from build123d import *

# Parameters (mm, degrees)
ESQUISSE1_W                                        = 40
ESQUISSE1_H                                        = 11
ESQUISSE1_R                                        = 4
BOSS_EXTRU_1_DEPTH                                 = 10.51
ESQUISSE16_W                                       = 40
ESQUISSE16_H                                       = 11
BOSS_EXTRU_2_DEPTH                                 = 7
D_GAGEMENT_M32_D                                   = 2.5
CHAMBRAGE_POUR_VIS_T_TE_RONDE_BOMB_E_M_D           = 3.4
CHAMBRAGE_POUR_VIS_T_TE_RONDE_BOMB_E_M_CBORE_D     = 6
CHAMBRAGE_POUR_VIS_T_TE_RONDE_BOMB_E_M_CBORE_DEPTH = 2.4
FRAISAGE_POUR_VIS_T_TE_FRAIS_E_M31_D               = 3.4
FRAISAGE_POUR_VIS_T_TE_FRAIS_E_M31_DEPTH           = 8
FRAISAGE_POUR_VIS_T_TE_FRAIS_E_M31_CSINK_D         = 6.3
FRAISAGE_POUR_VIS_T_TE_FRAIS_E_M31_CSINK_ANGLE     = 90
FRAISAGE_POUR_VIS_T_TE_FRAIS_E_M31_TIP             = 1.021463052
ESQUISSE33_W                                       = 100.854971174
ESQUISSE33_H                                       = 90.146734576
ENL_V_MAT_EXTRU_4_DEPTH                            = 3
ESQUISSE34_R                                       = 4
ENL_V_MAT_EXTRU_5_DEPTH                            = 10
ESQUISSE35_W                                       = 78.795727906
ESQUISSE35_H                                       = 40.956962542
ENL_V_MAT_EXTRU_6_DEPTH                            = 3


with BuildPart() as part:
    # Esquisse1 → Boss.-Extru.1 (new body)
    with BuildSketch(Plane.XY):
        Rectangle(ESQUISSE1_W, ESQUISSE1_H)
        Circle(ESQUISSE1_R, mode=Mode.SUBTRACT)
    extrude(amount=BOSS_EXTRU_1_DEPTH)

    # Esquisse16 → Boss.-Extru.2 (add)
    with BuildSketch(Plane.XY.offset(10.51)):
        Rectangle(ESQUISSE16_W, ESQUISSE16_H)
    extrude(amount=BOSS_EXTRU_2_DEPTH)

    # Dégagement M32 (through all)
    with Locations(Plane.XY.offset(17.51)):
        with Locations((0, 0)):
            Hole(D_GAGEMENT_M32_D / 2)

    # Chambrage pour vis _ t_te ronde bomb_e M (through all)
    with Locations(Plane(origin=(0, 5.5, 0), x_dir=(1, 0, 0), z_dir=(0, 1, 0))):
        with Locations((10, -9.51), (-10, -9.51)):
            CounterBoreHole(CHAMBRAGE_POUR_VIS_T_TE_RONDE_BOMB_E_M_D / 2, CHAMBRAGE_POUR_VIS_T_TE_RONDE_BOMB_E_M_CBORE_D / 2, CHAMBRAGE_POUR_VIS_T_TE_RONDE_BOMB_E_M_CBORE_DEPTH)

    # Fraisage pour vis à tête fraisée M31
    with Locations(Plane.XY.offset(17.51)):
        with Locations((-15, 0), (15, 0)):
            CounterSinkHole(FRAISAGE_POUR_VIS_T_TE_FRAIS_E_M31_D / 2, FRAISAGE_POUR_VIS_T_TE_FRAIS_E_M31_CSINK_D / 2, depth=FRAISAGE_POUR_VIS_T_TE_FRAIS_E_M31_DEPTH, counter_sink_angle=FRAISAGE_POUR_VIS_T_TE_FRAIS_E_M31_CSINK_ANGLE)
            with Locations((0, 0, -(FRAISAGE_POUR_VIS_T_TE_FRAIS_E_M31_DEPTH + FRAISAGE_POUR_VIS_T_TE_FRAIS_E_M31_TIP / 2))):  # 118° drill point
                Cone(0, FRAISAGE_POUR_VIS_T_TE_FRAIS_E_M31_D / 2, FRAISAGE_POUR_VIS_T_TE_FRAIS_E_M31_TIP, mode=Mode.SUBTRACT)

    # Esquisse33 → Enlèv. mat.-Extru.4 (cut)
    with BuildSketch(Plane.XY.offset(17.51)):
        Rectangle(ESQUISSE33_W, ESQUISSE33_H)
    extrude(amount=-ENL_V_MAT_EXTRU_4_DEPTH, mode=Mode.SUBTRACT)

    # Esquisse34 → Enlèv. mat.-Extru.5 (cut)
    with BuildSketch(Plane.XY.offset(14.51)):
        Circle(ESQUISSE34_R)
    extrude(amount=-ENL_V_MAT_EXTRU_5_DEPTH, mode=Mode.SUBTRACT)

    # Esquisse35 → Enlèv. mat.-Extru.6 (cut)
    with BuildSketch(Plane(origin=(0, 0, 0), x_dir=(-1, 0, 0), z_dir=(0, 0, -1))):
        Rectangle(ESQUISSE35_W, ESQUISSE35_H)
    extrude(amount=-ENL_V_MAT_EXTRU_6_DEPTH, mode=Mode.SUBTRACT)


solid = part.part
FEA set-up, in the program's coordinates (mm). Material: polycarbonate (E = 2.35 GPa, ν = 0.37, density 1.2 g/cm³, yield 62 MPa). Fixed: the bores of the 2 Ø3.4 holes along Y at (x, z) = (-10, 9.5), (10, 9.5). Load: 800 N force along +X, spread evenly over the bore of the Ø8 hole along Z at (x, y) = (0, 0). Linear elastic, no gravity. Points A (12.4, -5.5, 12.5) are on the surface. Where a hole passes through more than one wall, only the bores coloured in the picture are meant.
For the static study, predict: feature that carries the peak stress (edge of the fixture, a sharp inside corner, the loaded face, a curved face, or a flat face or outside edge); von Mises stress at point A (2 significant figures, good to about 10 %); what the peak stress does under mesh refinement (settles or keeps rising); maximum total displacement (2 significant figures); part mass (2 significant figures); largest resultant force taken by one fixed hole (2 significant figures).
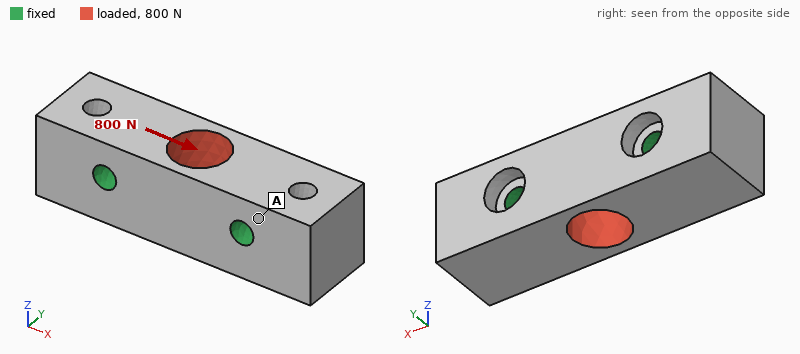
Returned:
edge of the fixture
1.5 MPa
keeps rising
24 µm
4.9 g
400 N
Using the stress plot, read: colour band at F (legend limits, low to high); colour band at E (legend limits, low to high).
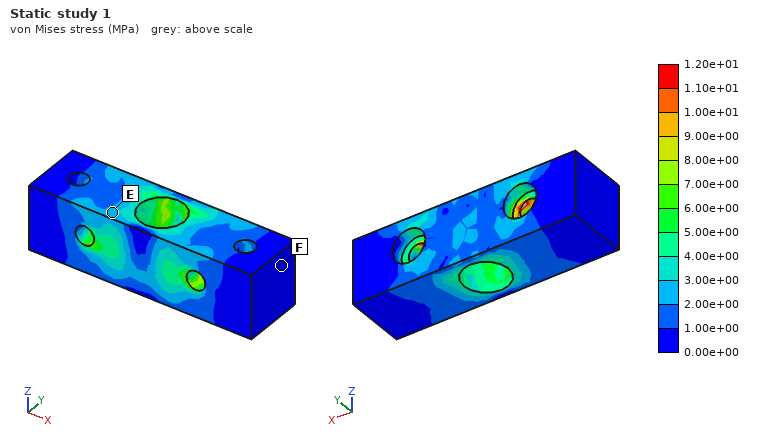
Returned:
0.00e+00 to 1.00e+00 MPa
2.00e+00 to 3.00e+00 MPa
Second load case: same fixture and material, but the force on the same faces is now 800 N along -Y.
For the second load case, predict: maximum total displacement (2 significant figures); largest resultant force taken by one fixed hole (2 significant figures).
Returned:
76 µm
400 N
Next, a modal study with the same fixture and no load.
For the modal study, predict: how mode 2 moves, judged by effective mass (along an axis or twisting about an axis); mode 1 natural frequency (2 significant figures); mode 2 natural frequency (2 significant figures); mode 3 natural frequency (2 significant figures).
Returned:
twisting about Y
9800 Hz
11 kHz
12 kHz
